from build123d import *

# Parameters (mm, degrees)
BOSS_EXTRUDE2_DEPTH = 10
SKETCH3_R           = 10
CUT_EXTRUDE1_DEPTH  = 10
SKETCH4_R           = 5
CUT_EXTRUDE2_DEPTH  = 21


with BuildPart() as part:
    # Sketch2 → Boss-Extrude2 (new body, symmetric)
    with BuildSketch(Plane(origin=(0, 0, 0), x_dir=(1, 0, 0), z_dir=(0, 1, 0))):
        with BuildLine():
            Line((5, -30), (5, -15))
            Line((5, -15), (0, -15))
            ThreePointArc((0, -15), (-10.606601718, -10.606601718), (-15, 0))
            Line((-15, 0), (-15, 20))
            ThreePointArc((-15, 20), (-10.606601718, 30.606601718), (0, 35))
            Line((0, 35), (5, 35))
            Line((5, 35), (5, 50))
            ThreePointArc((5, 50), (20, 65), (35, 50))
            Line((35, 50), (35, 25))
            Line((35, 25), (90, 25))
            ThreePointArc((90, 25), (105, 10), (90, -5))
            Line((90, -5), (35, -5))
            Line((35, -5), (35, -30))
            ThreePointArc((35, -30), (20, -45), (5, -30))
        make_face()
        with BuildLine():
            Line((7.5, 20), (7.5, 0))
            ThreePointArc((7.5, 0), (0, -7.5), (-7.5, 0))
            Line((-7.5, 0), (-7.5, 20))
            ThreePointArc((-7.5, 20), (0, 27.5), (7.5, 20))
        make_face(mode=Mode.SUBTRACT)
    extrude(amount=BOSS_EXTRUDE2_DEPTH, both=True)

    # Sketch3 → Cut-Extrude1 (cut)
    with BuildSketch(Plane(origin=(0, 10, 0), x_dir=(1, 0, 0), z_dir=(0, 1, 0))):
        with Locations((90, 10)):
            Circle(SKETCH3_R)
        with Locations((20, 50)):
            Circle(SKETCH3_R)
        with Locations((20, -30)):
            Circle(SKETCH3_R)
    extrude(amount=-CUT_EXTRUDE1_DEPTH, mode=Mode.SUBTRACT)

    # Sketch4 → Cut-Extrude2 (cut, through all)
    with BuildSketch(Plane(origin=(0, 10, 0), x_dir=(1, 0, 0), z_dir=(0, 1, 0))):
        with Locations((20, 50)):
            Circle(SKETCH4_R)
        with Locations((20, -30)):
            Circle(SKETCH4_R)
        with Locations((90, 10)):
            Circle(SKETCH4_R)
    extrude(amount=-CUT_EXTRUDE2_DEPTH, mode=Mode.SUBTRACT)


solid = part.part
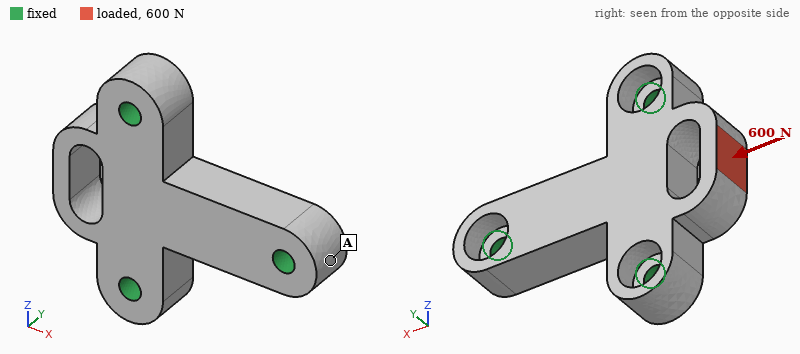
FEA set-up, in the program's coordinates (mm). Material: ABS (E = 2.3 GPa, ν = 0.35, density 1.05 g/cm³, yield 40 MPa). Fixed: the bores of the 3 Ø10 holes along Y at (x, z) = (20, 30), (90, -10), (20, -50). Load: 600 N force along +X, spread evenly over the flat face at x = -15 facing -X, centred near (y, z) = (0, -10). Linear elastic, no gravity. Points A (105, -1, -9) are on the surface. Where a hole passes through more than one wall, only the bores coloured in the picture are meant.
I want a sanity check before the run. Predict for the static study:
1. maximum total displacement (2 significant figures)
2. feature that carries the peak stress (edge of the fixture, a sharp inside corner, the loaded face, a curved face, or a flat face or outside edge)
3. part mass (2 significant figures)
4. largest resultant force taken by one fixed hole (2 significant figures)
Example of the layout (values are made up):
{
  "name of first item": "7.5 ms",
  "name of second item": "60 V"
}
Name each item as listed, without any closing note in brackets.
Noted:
{
  "maximum total displacement": "0.19 mm",
  "feature that carries the peak stress": "a curved face",
  "part mass": "100 g",
  "largest resultant force taken by one fixed hole": "250 N"
}
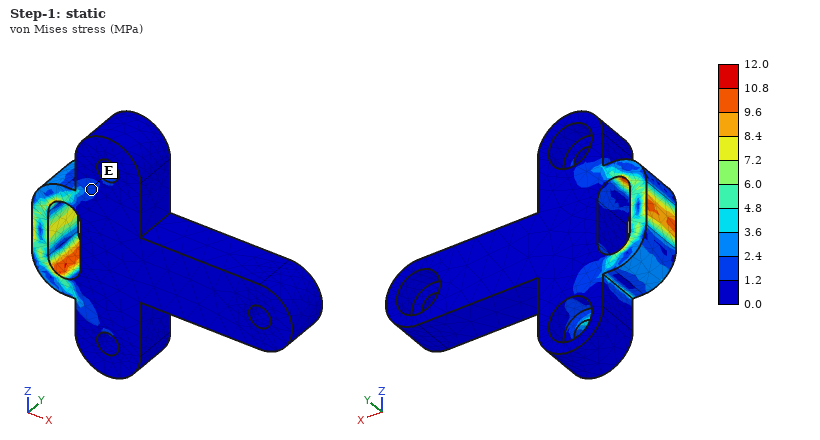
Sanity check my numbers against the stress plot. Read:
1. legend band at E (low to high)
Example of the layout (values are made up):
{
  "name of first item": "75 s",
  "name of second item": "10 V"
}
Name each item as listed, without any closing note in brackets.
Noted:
{
  "legend band at E": "1.2 to 2.4 MPa"
}
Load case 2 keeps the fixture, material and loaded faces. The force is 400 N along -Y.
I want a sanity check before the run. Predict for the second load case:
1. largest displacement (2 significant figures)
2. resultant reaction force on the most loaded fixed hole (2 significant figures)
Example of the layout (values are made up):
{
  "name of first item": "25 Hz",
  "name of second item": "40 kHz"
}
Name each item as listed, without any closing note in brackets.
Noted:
{
  "largest displacement": "0.44 mm",
  "resultant reaction force on the most loaded fixed hole": "330 N"
}
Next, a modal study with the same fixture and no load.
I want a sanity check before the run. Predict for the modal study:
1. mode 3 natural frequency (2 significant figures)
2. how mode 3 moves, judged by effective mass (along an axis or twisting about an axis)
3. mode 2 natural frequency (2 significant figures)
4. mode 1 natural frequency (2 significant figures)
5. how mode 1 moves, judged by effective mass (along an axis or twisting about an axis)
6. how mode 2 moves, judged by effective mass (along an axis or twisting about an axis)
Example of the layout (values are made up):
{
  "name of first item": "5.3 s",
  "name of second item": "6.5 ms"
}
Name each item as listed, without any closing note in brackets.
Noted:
{
  "mode 3 natural frequency": "3500 Hz",
  "how mode 3 moves, judged by effective mass": "along Z",
  "mode 2 natural frequency": "2600 Hz",
  "mode 1 natural frequency": "1900 Hz",
  "how mode 1 moves, judged by effective mass": "along Y",
  "how mode 2 moves, judged by effective mass": "along Y"
}
